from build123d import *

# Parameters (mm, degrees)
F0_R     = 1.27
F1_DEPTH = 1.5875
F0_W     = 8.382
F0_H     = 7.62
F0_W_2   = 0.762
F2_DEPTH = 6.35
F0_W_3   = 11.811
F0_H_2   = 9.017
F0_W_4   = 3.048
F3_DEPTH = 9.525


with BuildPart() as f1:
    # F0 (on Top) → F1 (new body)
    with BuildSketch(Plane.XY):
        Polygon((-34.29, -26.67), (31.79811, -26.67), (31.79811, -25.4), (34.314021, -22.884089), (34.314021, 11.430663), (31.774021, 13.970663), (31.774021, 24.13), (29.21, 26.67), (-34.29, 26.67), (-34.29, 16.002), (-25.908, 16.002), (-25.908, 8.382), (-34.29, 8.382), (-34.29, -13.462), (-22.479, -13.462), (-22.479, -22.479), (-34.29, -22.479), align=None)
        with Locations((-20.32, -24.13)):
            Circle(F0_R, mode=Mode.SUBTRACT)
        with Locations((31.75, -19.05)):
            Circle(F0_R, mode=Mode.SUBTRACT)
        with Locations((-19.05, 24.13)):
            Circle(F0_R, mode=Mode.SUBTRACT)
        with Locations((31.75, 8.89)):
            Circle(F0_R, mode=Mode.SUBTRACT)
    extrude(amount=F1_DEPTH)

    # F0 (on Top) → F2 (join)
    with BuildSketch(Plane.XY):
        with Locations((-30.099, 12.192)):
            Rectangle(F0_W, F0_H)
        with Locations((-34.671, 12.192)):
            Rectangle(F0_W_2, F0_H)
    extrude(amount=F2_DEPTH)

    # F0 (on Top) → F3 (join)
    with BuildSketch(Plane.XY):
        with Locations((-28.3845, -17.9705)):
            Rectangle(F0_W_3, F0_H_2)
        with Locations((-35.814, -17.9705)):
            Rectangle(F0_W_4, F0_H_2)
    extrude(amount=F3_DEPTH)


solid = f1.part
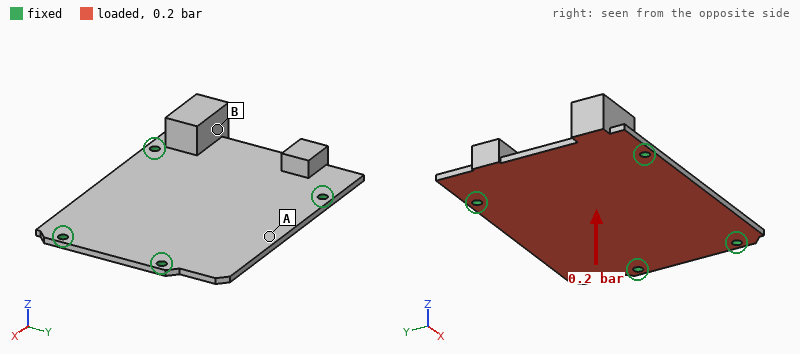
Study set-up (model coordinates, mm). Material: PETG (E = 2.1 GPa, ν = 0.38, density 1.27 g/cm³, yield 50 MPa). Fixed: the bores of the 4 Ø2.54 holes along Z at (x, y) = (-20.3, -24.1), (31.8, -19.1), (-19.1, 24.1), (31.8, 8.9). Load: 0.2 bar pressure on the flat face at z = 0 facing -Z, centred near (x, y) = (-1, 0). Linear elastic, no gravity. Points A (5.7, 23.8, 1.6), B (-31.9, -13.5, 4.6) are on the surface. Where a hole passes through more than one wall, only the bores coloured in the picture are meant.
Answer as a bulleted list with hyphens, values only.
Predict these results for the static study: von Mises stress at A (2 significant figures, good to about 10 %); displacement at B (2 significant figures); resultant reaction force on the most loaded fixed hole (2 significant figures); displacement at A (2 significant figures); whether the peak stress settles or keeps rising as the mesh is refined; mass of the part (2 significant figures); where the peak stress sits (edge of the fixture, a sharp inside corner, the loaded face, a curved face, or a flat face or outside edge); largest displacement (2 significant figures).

- 7.0 MPa
- 0.38 mm
- 22 N
- 0.79 mm
- keeps rising
- 9.1 g
- edge of the fixture
- 0.86 mm
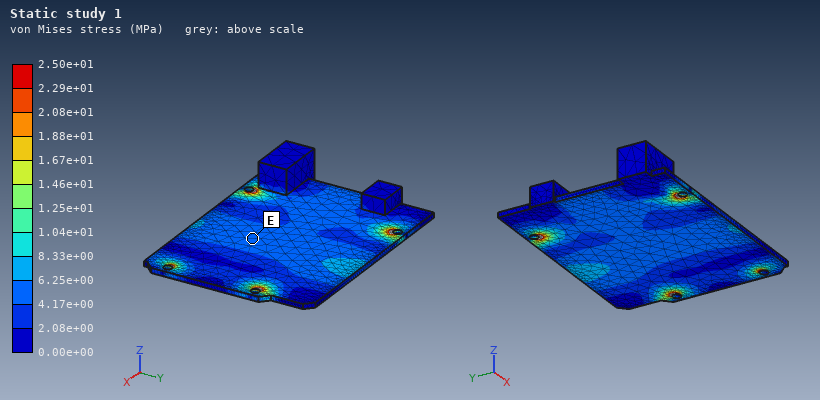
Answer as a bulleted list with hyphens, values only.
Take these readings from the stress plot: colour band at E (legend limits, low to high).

- 4.17e+00 to 6.25e+00 MPa
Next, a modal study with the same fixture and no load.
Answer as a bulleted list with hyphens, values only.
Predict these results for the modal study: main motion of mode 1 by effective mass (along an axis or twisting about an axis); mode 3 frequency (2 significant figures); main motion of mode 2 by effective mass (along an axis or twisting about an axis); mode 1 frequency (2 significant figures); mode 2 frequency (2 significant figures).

- along Z
- 760 Hz
- along Z
- 510 Hz
- 620 Hz
